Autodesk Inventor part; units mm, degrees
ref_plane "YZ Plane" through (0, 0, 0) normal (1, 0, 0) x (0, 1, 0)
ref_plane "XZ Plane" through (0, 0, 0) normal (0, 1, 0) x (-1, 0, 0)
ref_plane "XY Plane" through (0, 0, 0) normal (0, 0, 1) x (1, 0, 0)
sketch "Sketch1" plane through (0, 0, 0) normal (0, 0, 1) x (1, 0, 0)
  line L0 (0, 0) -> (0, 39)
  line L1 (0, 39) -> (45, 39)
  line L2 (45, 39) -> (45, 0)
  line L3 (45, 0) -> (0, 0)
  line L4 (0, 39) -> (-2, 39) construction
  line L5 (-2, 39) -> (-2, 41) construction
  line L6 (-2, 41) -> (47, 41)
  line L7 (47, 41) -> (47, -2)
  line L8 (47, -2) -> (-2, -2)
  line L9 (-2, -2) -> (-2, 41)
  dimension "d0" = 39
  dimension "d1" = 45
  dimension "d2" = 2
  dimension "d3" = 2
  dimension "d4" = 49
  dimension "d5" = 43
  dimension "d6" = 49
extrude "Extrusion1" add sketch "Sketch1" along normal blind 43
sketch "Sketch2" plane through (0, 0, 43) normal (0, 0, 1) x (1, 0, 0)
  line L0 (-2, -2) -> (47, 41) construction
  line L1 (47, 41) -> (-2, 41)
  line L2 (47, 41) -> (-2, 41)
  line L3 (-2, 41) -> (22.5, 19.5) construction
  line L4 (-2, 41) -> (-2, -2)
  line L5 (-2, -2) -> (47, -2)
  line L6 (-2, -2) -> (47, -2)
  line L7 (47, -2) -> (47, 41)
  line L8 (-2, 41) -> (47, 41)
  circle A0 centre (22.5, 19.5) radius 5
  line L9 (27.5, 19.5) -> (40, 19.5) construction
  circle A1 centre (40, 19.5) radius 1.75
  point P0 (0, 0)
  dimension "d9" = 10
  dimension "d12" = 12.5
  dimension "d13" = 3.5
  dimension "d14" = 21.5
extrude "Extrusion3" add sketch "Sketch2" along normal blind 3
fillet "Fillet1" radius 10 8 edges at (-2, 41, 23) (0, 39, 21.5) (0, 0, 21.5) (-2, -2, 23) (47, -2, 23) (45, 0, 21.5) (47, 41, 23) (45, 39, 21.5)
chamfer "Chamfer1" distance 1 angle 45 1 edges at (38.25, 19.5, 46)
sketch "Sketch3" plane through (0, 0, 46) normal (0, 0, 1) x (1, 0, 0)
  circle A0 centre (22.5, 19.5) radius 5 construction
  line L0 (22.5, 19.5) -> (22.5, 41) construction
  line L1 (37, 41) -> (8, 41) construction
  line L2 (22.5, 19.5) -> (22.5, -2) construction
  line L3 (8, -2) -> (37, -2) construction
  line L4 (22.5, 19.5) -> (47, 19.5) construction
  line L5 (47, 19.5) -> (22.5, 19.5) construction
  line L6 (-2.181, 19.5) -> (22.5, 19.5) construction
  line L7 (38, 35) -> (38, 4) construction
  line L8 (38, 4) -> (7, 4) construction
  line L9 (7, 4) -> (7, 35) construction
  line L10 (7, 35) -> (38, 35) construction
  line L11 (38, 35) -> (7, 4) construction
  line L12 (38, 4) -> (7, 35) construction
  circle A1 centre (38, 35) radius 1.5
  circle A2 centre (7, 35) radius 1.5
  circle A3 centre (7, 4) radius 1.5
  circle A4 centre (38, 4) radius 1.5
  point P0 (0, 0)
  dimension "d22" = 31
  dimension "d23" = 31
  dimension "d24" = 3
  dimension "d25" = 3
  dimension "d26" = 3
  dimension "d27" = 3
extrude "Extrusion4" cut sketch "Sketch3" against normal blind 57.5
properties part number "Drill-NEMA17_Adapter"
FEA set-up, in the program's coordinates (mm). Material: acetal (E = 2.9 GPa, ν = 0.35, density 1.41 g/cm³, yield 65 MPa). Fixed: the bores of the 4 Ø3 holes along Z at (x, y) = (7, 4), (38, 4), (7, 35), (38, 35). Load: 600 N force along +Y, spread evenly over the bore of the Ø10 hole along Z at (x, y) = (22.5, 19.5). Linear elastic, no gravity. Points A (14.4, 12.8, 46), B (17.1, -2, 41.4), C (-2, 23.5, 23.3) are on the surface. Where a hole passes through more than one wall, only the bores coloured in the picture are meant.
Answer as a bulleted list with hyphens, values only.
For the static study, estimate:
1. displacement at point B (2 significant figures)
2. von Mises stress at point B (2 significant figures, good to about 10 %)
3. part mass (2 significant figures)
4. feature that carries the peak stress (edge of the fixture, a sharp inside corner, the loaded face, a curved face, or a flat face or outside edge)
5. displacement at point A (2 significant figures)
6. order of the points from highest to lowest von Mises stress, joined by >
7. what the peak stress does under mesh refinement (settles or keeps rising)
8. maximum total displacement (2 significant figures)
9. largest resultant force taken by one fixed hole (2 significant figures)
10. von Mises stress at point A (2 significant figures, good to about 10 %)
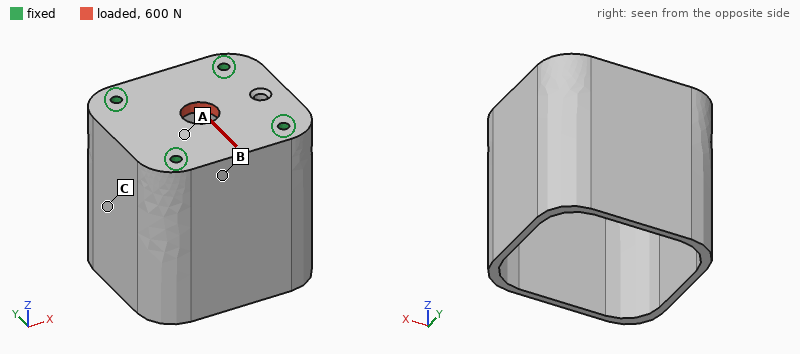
- 23 µm
- 2.0 MPa
- 29 g
- edge of the fixture
- 24 µm
- A > B > C
- keeps rising
- 44 µm
- 160 N
- 4.8 MPa
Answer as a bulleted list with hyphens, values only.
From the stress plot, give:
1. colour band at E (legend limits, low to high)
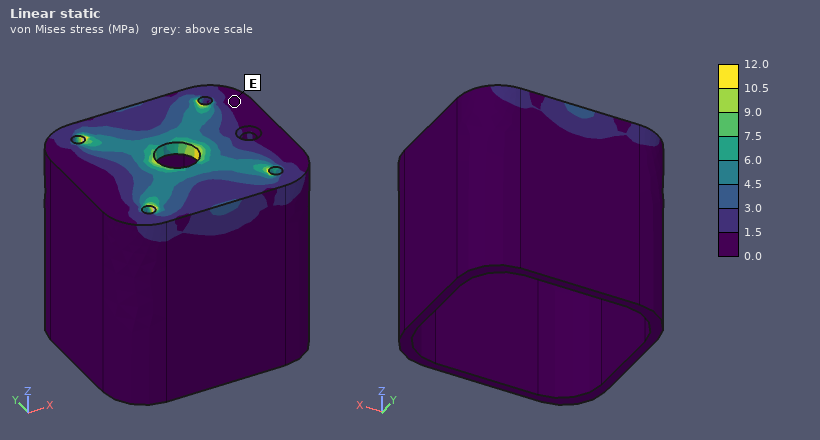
- 0.0 to 1.5 MPa
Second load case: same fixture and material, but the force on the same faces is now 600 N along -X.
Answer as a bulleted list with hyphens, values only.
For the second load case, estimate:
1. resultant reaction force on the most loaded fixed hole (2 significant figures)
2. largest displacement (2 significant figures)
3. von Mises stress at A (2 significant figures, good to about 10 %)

- 160 N
- 41 µm
- 4.7 MPa
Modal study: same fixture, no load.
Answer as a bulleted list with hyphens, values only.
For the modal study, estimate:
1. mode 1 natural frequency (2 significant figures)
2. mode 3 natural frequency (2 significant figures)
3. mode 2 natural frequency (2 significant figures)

- 940 Hz
- 1500 Hz
- 1400 Hz
